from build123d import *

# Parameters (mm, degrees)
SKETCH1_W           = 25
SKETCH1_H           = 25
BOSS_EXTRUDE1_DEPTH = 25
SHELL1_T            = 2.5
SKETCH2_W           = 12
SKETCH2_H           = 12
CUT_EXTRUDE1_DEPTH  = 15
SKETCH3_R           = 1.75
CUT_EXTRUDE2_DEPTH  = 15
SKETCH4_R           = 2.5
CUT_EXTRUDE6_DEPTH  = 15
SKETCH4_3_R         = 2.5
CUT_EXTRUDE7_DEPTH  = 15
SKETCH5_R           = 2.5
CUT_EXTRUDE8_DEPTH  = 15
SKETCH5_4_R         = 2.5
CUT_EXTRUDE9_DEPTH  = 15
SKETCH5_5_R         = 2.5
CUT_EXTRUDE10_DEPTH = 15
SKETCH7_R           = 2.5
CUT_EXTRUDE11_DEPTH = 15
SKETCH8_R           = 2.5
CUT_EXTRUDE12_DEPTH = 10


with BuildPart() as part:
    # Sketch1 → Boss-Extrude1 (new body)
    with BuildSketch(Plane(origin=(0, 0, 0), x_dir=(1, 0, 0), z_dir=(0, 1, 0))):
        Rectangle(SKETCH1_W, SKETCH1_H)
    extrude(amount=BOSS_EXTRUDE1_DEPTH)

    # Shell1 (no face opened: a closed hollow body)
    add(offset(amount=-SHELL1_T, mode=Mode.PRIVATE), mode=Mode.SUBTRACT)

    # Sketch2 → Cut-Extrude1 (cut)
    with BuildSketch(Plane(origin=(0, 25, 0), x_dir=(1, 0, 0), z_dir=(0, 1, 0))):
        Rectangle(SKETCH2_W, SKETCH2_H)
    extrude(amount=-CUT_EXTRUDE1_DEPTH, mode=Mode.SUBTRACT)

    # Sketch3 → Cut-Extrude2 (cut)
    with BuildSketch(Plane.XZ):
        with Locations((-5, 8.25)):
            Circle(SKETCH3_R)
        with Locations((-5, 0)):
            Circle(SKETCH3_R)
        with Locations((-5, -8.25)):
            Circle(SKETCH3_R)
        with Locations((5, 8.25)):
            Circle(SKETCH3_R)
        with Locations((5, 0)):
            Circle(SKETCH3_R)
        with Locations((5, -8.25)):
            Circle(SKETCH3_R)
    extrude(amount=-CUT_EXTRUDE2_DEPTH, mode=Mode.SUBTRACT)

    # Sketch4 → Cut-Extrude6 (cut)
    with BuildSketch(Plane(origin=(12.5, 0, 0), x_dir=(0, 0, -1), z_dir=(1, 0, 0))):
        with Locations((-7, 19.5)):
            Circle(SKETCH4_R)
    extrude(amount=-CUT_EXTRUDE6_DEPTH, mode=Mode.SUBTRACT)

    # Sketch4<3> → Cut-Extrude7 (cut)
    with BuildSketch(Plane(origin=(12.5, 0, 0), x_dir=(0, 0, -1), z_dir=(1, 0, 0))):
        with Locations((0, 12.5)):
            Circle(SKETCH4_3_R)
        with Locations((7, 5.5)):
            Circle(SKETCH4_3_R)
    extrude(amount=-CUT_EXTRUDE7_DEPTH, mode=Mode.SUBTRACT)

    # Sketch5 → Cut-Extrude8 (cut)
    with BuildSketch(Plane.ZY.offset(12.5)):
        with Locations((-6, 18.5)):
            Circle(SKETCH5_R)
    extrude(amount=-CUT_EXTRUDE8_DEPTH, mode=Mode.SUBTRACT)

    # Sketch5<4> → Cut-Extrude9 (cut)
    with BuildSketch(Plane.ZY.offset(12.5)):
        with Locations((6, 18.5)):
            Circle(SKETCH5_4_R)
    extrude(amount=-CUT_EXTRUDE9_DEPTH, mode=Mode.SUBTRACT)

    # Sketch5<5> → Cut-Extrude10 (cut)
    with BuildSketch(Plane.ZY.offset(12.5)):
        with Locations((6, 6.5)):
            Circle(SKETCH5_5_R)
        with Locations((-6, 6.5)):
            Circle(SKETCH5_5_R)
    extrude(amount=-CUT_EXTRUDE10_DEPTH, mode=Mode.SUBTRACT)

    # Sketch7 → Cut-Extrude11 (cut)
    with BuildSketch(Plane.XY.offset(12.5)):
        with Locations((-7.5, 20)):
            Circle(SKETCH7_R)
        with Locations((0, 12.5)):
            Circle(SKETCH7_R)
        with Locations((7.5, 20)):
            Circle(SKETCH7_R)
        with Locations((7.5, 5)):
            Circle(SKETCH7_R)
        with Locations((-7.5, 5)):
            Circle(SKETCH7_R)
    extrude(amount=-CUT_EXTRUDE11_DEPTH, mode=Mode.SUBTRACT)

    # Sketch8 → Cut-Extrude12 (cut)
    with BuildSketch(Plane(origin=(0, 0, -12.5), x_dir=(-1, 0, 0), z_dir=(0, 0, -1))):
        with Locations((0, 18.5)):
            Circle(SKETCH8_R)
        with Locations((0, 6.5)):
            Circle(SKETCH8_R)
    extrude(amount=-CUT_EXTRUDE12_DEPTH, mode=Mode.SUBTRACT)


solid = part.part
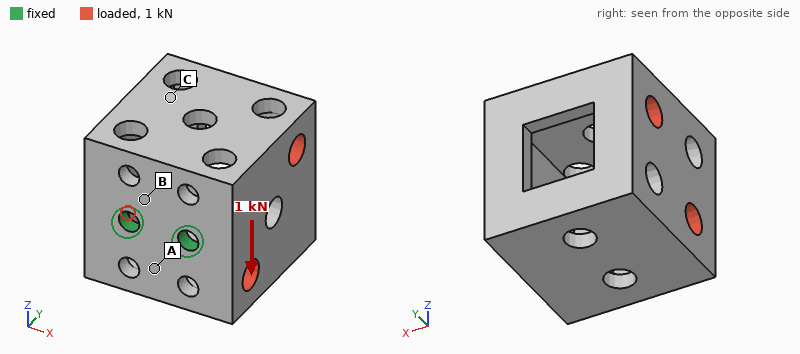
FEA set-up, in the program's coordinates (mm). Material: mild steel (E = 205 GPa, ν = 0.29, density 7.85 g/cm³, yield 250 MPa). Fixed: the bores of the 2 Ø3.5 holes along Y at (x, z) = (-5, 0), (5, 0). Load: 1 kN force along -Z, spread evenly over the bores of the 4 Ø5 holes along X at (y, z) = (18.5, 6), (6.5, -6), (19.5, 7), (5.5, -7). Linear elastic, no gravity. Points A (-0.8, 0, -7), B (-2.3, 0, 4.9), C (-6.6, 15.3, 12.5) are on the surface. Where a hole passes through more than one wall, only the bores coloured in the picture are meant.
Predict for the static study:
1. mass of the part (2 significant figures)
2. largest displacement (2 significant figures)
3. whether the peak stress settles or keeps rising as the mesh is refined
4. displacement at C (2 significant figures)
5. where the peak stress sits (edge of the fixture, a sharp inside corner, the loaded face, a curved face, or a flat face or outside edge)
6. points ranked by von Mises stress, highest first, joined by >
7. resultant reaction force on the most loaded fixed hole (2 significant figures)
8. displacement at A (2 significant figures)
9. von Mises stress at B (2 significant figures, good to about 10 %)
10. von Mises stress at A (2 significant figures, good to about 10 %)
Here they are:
51 g
68 µm
keeps rising
48 µm
edge of the fixture
B > A > C
500 N
13 µm
85 MPa
57 MPa
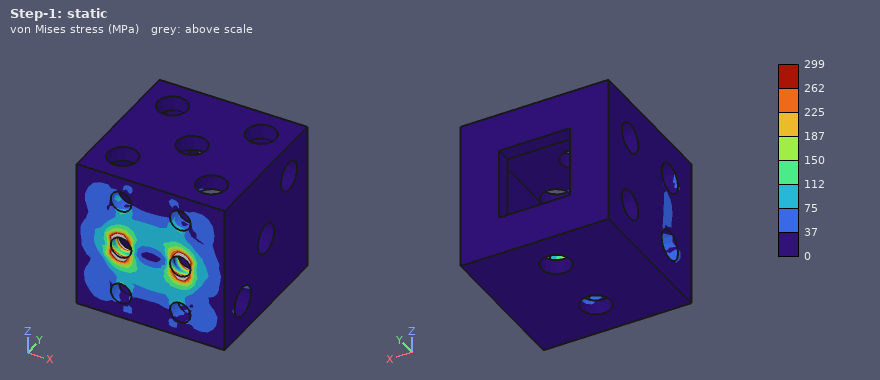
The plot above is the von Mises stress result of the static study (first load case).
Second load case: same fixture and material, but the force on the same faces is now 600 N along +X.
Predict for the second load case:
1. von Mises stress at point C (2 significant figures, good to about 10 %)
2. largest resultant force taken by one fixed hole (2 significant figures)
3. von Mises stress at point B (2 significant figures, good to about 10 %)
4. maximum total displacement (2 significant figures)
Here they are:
11 MPa
500 N
12 MPa
16 µm
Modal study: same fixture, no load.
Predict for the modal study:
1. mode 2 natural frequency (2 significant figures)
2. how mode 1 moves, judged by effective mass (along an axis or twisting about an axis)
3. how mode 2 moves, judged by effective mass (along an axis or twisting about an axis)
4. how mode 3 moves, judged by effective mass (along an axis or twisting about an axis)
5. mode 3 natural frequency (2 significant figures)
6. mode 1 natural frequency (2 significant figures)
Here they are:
4900 Hz
along Z
along X
along Y
11 kHz
2900 Hz
